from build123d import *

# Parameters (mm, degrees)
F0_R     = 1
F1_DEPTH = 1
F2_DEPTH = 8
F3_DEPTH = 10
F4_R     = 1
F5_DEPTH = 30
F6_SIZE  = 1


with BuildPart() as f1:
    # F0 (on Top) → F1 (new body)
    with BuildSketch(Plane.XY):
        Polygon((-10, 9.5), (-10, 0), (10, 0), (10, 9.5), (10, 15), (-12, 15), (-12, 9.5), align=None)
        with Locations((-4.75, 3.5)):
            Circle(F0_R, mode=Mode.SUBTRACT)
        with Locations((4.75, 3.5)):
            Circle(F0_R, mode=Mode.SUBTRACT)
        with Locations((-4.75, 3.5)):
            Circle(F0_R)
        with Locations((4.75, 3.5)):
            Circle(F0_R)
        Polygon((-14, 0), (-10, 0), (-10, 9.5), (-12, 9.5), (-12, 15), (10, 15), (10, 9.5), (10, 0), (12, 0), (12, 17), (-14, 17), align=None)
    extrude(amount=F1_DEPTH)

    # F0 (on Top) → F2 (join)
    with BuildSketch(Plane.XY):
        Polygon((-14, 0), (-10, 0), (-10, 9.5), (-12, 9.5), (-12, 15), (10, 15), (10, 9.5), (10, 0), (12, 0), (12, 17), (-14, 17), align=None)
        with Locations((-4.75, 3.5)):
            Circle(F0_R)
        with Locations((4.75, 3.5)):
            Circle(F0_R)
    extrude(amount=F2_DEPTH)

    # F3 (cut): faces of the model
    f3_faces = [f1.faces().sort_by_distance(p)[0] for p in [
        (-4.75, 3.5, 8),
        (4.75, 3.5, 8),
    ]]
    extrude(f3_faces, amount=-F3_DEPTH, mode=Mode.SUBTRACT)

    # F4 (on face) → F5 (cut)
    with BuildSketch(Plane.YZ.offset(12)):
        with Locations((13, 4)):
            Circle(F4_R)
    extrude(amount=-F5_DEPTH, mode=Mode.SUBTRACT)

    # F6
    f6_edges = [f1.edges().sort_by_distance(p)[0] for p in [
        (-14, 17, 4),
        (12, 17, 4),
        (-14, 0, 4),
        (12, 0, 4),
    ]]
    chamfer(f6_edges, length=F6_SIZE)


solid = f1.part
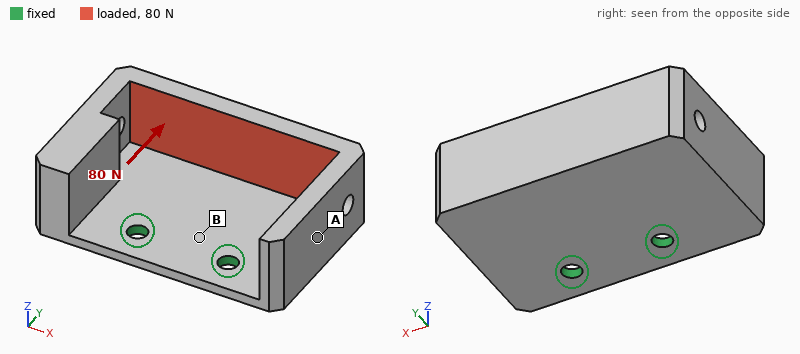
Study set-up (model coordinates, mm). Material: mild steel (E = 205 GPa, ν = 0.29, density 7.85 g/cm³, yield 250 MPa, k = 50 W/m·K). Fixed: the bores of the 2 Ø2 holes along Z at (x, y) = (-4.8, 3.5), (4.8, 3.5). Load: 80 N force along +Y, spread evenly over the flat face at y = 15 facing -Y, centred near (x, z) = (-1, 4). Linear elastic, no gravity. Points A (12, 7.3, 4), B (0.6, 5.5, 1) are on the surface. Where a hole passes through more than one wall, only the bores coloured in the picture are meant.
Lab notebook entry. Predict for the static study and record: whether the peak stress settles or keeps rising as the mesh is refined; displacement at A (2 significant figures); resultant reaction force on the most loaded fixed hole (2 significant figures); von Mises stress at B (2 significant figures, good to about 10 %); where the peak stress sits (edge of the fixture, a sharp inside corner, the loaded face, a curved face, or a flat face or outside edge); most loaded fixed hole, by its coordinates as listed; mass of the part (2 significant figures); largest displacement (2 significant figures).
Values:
keeps rising
8.5 µm
47 N
36 MPa
edge of the fixture
(-4.8, 3.5)
10 g
31 µm
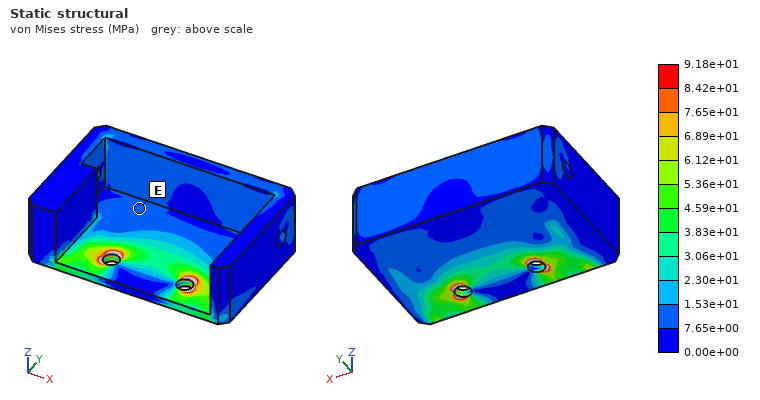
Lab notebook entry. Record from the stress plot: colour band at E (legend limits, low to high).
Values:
7.65e+00 to 1.53e+01 MPa
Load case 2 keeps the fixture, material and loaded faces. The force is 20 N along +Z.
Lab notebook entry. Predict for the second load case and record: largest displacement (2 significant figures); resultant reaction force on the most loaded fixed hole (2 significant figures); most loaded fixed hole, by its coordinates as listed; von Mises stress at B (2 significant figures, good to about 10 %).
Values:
20 µm
11 N
(-4.8, 3.5)
26 MPa
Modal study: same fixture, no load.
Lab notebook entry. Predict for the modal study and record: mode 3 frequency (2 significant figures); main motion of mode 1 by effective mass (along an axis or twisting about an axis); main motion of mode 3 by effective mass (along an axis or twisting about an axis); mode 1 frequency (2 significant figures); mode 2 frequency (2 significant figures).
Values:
8300 Hz
along Z
along Z
2300 Hz
3000 Hz
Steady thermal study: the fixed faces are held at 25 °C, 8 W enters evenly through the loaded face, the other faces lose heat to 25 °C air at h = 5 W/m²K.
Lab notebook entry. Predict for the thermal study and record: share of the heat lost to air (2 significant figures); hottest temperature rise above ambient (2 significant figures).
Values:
4.3 %
74 K
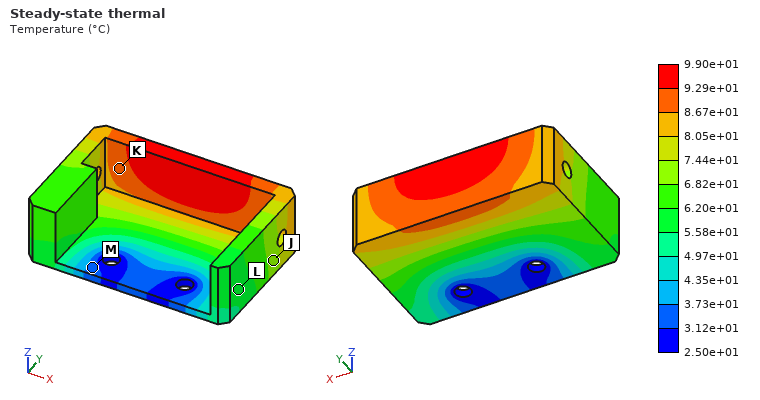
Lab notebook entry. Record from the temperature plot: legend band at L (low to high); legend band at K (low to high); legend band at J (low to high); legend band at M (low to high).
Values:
5.58e+01 to 6.20e+01 °C
8.67e+01 to 9.29e+01 °C
6.82e+01 to 7.44e+01 °C
3.12e+01 to 3.73e+01 °C
